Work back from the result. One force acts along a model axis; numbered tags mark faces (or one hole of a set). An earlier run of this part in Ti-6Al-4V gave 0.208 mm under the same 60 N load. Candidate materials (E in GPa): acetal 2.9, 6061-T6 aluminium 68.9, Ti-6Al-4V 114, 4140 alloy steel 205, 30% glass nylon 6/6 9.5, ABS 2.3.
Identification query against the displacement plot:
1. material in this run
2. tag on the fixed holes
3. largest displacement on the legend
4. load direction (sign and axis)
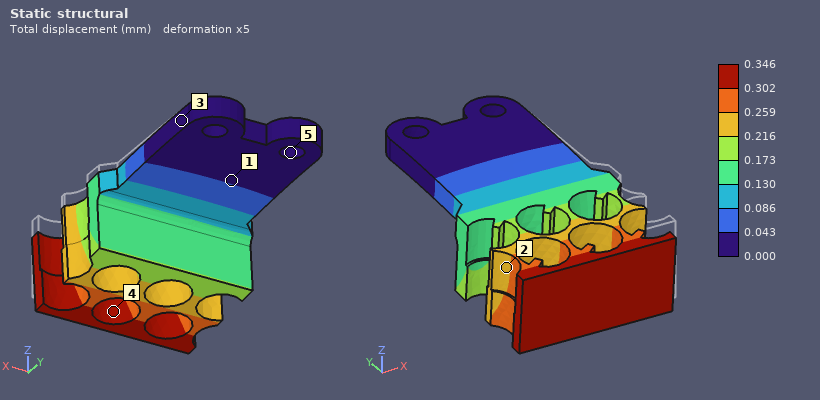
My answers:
6061-T6 aluminium
5
0.346 mm
-Z
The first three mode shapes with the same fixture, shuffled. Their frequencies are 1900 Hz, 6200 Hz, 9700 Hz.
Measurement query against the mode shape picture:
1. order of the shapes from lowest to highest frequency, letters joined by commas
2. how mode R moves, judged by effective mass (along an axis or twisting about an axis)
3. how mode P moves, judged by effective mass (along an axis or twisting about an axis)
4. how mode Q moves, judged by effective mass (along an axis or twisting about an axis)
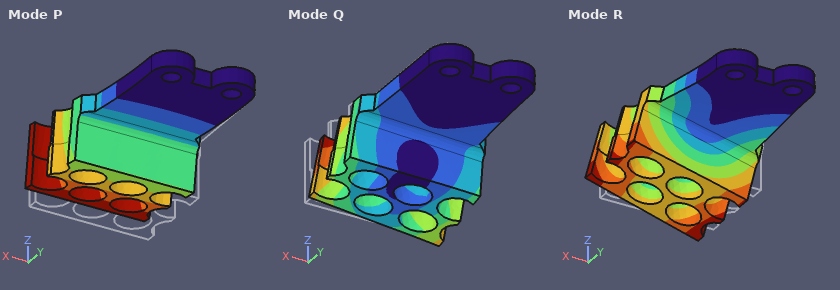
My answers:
P, R, Q
along X
along Z
along X
